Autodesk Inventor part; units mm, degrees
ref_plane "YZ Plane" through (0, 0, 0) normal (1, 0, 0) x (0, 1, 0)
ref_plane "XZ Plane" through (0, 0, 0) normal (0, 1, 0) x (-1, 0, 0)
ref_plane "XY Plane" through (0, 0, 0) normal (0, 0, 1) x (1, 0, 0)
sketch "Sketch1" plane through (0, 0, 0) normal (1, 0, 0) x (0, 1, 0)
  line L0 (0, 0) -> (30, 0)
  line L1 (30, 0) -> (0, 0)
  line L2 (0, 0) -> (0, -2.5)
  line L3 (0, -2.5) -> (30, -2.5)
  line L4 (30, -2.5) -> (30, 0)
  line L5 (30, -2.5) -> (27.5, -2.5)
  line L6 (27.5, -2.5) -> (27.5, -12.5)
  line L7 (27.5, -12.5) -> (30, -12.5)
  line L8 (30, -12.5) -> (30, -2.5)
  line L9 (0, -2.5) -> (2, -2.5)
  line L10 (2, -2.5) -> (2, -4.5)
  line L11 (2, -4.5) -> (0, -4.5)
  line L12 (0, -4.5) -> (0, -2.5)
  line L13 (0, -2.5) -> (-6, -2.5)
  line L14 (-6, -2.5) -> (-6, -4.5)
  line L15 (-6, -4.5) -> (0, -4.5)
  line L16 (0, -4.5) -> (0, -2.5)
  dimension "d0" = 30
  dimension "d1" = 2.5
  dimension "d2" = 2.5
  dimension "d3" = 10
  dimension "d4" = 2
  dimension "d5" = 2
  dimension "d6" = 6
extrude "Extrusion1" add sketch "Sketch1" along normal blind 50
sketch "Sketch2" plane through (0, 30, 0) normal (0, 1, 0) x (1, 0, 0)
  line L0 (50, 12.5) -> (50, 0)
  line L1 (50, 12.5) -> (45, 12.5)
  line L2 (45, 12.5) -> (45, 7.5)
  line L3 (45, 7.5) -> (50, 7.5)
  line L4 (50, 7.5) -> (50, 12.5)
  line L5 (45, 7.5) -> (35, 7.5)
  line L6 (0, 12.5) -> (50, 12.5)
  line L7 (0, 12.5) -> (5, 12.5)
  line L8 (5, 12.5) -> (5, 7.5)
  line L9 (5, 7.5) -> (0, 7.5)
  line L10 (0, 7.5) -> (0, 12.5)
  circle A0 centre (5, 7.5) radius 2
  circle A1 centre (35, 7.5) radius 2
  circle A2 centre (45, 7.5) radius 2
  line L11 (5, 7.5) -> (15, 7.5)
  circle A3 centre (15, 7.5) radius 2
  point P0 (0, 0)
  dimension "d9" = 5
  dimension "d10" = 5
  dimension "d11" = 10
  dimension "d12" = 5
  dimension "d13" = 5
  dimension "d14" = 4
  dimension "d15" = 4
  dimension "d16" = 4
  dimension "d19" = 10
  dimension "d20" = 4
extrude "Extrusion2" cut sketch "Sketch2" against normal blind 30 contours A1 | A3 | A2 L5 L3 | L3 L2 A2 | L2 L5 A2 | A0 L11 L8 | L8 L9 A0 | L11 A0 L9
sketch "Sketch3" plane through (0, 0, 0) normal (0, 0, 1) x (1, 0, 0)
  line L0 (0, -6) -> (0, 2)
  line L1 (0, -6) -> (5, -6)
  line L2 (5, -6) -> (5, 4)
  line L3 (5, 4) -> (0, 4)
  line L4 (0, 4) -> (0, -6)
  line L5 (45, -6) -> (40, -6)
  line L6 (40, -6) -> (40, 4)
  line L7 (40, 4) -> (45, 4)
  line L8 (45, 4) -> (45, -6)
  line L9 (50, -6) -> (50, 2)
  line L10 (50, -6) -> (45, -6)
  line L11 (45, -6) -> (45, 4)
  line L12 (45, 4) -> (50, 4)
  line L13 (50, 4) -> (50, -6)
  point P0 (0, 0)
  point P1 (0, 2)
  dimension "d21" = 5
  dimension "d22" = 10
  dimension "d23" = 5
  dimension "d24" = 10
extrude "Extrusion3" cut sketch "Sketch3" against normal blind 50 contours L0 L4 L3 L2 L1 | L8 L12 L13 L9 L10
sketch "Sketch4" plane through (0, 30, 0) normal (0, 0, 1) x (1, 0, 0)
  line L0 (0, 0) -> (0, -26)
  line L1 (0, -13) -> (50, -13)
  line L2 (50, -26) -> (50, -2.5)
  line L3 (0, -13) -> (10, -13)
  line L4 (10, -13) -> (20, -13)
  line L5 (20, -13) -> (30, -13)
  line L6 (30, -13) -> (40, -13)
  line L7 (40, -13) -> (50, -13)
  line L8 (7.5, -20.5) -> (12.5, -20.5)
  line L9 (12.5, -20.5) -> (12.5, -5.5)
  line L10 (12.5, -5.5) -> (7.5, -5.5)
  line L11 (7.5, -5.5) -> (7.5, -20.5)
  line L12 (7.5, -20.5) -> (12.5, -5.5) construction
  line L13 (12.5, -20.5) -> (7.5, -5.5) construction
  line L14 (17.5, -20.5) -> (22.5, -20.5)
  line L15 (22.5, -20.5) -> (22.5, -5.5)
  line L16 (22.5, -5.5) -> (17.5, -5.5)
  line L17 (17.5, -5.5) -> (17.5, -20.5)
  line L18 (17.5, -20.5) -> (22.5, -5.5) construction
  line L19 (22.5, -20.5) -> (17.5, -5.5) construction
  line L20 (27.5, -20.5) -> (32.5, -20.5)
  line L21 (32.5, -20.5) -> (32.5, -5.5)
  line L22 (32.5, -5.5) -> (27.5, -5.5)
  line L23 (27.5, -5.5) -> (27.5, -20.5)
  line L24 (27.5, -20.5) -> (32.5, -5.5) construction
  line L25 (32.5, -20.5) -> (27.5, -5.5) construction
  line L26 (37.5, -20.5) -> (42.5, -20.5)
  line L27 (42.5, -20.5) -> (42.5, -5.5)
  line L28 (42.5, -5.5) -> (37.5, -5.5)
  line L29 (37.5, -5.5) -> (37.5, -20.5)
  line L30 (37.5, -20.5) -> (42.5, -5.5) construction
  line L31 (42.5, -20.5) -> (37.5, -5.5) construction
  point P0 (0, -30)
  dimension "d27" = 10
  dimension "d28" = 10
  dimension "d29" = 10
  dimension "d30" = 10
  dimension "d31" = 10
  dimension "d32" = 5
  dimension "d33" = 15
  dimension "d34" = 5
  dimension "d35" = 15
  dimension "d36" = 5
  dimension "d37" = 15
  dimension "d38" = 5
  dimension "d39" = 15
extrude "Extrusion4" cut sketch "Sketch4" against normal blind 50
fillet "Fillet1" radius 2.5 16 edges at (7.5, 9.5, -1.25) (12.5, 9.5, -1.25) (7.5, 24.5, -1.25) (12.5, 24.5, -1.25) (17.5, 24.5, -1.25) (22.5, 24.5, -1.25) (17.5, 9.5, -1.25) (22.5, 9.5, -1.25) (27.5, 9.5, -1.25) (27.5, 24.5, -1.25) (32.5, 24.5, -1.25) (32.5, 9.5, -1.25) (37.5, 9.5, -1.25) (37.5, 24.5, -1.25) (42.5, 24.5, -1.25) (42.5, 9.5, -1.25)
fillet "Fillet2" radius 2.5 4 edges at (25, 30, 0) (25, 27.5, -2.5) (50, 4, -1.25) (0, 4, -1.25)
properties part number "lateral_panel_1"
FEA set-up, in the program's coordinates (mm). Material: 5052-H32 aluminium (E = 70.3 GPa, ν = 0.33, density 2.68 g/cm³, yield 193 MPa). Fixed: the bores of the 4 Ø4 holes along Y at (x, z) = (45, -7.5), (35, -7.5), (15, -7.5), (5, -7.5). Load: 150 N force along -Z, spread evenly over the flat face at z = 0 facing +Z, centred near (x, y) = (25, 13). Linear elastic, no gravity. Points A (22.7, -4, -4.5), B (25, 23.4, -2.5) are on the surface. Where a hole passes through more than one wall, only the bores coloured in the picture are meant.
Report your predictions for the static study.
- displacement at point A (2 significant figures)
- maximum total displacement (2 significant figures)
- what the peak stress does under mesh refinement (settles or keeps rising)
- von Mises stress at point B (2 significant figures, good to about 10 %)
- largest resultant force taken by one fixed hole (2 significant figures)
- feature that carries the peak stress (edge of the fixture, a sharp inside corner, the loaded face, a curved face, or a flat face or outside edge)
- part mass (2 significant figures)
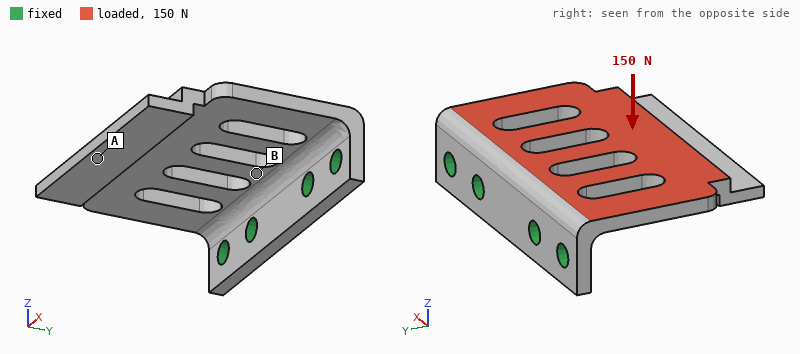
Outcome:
0.21 mm
0.23 mm
keeps rising
46 MPa
45 N
edge of the fixture
13 g
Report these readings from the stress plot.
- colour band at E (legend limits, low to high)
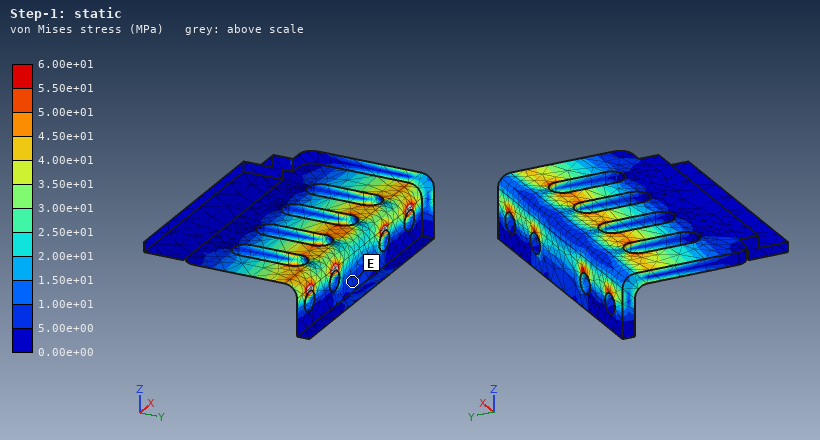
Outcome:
5.00e+00 to 1.00e+01 MPa
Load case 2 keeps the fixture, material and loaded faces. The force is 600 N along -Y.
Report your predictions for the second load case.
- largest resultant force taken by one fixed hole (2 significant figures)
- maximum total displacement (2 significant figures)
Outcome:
160 N
0.16 mm
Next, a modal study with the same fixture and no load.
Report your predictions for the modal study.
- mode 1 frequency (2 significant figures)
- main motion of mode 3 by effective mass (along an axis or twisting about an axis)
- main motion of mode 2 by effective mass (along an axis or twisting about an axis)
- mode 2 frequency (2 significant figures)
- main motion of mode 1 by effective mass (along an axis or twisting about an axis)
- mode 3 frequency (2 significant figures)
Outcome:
1500 Hz
along X
twisting about Y
3200 Hz
along Z
7800 Hz
